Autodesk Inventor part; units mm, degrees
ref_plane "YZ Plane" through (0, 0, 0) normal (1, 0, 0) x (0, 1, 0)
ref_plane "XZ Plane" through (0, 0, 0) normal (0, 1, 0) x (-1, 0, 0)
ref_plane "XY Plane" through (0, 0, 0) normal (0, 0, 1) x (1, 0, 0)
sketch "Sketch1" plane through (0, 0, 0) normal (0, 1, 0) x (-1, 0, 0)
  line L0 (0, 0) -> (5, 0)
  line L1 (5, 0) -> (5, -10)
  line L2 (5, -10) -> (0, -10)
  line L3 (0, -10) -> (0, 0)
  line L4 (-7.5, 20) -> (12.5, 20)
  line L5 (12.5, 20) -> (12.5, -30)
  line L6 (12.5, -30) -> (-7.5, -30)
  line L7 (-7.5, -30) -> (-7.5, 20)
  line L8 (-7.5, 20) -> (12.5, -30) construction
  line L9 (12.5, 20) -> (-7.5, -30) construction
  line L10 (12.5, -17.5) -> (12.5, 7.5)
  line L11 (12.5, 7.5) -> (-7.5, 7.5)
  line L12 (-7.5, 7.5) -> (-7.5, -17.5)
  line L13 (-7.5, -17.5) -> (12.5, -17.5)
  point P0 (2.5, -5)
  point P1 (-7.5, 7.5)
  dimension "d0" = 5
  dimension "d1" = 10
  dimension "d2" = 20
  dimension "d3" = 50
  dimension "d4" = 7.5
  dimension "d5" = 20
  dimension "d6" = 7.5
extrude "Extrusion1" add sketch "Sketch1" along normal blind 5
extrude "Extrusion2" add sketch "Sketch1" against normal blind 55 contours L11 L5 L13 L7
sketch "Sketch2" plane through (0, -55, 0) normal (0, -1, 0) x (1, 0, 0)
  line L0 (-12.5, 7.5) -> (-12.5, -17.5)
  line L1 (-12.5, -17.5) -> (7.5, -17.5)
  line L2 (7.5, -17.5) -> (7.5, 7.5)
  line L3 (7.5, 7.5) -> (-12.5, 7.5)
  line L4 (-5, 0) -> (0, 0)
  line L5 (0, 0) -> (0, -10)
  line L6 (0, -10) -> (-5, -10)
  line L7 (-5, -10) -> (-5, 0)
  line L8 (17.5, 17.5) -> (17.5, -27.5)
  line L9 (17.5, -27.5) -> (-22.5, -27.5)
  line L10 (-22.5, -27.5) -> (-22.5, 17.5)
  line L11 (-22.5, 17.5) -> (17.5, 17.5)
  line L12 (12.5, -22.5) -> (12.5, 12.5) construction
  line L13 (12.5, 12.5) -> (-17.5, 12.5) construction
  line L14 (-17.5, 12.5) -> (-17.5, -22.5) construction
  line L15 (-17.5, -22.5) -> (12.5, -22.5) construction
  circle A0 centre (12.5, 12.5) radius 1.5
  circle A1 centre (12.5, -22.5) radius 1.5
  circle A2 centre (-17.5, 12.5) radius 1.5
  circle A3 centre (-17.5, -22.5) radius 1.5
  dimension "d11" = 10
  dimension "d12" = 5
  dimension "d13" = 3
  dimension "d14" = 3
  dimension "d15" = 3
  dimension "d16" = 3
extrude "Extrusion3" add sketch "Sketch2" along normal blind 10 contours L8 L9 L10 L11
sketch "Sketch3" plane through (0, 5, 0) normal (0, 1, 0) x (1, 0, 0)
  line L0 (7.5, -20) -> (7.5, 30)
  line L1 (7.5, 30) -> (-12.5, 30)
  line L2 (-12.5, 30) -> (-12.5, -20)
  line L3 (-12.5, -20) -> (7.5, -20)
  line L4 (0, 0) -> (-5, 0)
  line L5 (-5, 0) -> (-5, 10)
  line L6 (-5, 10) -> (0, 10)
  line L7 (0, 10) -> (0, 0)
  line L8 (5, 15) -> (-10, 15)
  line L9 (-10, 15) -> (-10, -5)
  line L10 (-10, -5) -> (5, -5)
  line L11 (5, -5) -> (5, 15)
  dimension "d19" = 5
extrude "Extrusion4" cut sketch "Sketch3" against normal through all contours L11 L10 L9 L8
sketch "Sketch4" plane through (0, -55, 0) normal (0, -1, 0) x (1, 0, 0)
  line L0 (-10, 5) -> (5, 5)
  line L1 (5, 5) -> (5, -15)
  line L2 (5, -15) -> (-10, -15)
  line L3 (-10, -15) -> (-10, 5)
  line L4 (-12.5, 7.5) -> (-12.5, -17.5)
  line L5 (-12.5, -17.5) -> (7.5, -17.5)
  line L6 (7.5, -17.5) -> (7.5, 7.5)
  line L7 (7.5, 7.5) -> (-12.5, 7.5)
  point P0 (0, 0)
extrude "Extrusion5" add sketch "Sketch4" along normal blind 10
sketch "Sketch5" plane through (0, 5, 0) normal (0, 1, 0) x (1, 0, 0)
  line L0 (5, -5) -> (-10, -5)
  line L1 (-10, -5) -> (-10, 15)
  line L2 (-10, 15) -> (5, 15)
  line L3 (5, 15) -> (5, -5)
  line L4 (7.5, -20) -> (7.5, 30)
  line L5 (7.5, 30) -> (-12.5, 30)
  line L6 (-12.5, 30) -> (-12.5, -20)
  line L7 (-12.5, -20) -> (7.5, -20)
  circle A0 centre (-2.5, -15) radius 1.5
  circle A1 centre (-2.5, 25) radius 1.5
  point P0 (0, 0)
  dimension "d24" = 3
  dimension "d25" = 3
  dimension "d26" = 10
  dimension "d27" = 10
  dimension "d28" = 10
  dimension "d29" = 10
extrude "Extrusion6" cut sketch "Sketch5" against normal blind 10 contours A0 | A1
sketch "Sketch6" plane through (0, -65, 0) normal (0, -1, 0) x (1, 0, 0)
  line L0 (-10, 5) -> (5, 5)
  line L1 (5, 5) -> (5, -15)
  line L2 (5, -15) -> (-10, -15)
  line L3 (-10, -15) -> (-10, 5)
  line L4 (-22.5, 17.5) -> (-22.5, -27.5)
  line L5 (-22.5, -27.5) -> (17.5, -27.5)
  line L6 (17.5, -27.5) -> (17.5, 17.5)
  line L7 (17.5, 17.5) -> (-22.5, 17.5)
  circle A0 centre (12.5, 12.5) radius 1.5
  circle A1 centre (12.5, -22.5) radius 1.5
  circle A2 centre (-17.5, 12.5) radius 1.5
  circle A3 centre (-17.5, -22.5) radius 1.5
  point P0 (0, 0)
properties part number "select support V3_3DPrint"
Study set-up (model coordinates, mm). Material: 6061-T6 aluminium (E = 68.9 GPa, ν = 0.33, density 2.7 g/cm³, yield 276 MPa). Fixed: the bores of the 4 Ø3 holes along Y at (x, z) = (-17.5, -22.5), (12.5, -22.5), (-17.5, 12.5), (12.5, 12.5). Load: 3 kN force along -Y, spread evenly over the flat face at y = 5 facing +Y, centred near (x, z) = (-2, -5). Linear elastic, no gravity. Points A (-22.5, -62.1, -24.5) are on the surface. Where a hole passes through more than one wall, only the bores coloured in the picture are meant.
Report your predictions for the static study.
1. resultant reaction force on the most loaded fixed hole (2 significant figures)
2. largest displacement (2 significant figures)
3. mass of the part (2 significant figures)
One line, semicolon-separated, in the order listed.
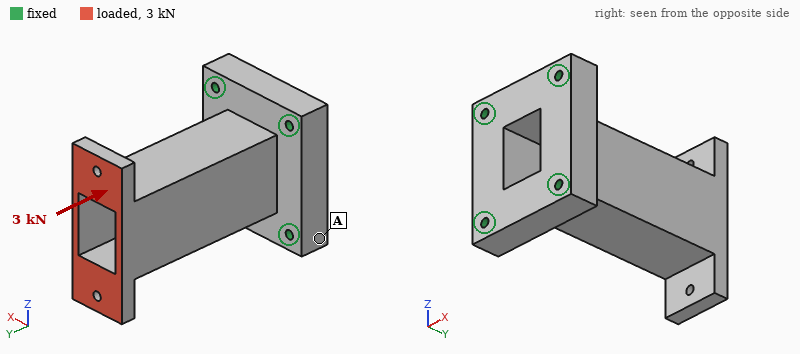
770 N; 0.10 mm; 79 g
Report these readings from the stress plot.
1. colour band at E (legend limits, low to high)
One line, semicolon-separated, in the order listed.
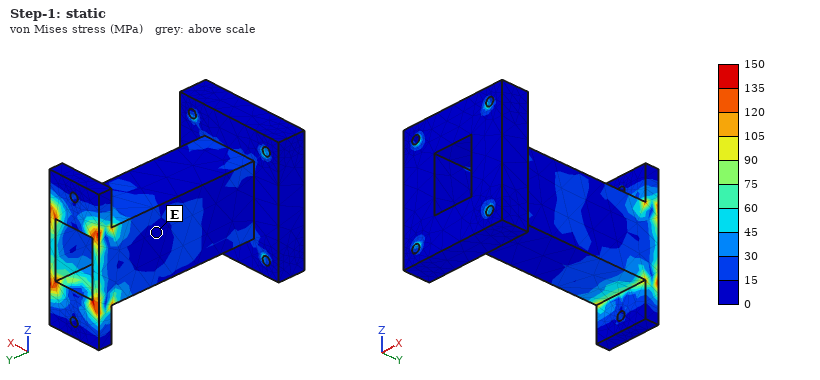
0 to 15 MPa
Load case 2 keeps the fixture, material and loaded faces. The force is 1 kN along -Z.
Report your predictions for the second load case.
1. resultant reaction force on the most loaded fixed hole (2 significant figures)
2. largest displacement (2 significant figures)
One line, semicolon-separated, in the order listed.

1.1 kN; 0.15 mm
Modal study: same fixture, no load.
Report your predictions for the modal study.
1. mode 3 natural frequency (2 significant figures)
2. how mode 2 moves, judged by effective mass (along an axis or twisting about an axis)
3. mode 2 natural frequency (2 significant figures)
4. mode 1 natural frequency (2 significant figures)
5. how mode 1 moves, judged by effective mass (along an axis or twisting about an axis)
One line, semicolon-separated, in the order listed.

7100 Hz; along Z; 3500 Hz; 3000 Hz; along X
